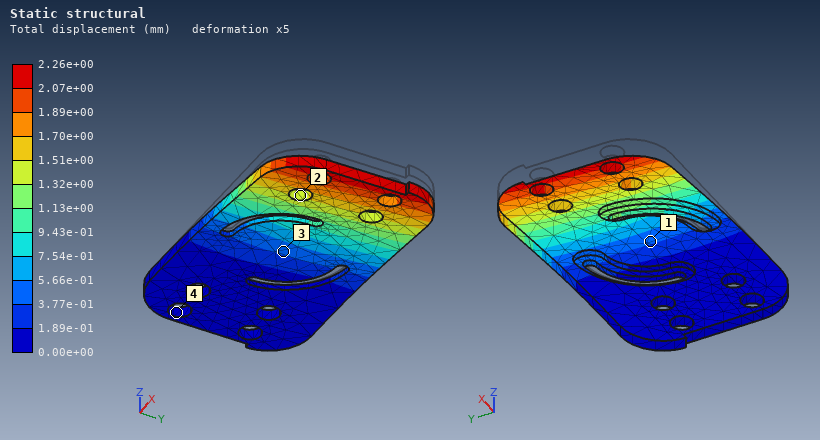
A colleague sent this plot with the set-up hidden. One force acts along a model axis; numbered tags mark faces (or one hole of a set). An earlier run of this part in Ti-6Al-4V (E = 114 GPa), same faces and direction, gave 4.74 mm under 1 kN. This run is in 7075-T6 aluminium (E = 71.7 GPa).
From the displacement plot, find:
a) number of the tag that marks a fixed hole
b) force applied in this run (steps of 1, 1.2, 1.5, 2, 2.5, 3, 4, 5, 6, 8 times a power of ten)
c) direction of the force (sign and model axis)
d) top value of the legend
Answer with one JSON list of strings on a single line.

["4", "300 N", "-Z", "2.26e+00 mm"]
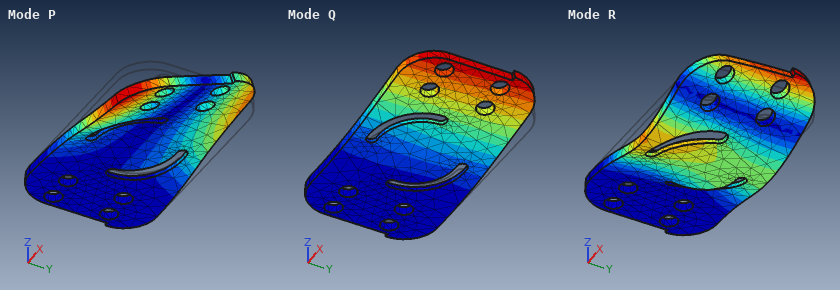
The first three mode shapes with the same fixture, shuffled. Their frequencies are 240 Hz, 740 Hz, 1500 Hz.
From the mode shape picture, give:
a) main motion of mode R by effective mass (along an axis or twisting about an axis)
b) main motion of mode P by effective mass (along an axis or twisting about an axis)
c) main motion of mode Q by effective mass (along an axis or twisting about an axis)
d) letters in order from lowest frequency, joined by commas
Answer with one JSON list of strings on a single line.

["along Z", "twisting about X", "along Z", "Q, P, R"]
